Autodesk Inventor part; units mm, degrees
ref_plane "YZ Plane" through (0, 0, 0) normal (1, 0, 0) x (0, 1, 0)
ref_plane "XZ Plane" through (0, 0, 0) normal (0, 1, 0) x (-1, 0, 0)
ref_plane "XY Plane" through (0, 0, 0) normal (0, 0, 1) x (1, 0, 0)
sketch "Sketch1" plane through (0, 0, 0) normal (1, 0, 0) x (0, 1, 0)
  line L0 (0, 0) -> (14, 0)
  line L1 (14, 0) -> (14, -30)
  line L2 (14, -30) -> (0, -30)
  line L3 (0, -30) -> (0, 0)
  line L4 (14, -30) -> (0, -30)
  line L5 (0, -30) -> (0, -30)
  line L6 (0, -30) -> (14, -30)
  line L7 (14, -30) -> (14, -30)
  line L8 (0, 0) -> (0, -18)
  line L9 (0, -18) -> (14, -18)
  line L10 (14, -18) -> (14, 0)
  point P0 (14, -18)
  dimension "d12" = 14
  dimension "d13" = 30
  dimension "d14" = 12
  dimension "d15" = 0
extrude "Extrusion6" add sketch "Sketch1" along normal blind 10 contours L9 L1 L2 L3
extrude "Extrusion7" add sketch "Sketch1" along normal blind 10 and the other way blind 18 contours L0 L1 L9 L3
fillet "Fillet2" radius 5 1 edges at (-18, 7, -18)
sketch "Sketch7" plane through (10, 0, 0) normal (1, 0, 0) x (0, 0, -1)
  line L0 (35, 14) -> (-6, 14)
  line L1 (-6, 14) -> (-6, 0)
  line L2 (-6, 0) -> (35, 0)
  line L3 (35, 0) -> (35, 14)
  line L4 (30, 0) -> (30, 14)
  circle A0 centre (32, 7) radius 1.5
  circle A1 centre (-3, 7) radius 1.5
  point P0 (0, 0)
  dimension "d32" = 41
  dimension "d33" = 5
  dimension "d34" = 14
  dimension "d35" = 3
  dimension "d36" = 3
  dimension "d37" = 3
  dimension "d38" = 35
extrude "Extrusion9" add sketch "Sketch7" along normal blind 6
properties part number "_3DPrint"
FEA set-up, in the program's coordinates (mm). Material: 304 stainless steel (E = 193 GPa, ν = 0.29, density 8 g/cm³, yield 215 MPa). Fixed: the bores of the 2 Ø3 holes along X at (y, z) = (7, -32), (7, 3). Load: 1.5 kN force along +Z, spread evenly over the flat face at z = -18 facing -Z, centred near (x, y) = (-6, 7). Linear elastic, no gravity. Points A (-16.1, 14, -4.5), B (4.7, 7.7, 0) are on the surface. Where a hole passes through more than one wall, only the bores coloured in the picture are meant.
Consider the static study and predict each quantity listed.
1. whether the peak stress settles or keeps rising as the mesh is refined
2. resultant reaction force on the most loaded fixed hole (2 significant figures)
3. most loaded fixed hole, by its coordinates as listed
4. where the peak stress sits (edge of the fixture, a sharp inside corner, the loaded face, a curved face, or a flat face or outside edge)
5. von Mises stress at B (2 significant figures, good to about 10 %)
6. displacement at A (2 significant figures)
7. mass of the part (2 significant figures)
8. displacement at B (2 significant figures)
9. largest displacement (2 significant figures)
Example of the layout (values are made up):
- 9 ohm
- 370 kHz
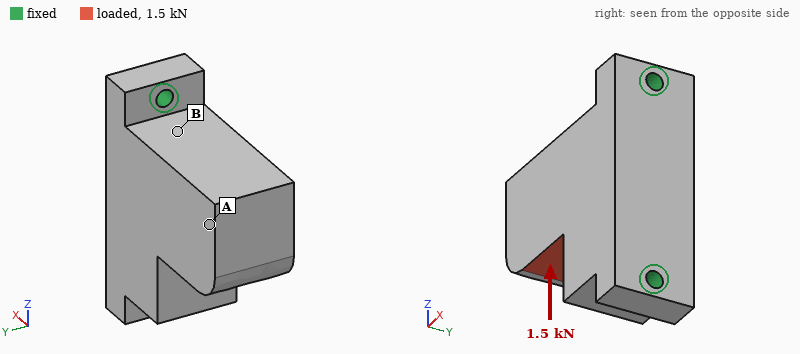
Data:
- keeps rising
- 1.3 kN
- (7, -32)
- edge of the fixture
- 15 MPa
- 5.8 µm
- 96 g
- 2.1 µm
- 6.4 µm
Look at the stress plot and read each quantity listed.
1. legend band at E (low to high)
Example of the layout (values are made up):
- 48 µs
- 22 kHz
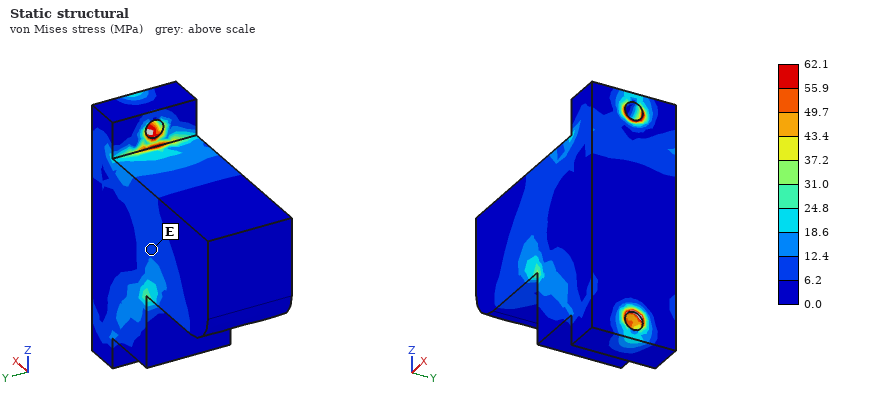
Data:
- 6.2 to 12.4 MPa
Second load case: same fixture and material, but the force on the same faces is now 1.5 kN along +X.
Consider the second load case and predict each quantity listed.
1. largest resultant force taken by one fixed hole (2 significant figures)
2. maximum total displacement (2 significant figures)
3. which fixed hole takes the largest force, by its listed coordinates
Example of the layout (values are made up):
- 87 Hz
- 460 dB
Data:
- 1.0 kN
- 4.4 µm
- (7, -32)
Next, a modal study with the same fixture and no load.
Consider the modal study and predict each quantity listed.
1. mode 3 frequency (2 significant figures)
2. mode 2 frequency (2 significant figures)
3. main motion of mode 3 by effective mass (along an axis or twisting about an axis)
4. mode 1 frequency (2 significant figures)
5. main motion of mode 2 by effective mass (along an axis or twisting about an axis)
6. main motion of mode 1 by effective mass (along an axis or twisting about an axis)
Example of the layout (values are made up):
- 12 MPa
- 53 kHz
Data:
- 17 kHz
- 13 kHz
- along X
- 4500 Hz
- along Z
- along Y
